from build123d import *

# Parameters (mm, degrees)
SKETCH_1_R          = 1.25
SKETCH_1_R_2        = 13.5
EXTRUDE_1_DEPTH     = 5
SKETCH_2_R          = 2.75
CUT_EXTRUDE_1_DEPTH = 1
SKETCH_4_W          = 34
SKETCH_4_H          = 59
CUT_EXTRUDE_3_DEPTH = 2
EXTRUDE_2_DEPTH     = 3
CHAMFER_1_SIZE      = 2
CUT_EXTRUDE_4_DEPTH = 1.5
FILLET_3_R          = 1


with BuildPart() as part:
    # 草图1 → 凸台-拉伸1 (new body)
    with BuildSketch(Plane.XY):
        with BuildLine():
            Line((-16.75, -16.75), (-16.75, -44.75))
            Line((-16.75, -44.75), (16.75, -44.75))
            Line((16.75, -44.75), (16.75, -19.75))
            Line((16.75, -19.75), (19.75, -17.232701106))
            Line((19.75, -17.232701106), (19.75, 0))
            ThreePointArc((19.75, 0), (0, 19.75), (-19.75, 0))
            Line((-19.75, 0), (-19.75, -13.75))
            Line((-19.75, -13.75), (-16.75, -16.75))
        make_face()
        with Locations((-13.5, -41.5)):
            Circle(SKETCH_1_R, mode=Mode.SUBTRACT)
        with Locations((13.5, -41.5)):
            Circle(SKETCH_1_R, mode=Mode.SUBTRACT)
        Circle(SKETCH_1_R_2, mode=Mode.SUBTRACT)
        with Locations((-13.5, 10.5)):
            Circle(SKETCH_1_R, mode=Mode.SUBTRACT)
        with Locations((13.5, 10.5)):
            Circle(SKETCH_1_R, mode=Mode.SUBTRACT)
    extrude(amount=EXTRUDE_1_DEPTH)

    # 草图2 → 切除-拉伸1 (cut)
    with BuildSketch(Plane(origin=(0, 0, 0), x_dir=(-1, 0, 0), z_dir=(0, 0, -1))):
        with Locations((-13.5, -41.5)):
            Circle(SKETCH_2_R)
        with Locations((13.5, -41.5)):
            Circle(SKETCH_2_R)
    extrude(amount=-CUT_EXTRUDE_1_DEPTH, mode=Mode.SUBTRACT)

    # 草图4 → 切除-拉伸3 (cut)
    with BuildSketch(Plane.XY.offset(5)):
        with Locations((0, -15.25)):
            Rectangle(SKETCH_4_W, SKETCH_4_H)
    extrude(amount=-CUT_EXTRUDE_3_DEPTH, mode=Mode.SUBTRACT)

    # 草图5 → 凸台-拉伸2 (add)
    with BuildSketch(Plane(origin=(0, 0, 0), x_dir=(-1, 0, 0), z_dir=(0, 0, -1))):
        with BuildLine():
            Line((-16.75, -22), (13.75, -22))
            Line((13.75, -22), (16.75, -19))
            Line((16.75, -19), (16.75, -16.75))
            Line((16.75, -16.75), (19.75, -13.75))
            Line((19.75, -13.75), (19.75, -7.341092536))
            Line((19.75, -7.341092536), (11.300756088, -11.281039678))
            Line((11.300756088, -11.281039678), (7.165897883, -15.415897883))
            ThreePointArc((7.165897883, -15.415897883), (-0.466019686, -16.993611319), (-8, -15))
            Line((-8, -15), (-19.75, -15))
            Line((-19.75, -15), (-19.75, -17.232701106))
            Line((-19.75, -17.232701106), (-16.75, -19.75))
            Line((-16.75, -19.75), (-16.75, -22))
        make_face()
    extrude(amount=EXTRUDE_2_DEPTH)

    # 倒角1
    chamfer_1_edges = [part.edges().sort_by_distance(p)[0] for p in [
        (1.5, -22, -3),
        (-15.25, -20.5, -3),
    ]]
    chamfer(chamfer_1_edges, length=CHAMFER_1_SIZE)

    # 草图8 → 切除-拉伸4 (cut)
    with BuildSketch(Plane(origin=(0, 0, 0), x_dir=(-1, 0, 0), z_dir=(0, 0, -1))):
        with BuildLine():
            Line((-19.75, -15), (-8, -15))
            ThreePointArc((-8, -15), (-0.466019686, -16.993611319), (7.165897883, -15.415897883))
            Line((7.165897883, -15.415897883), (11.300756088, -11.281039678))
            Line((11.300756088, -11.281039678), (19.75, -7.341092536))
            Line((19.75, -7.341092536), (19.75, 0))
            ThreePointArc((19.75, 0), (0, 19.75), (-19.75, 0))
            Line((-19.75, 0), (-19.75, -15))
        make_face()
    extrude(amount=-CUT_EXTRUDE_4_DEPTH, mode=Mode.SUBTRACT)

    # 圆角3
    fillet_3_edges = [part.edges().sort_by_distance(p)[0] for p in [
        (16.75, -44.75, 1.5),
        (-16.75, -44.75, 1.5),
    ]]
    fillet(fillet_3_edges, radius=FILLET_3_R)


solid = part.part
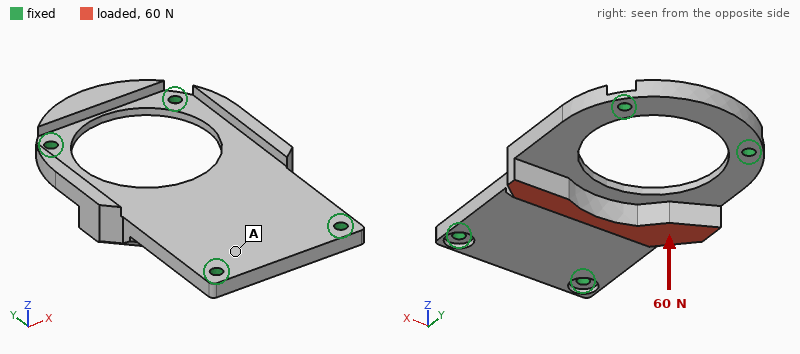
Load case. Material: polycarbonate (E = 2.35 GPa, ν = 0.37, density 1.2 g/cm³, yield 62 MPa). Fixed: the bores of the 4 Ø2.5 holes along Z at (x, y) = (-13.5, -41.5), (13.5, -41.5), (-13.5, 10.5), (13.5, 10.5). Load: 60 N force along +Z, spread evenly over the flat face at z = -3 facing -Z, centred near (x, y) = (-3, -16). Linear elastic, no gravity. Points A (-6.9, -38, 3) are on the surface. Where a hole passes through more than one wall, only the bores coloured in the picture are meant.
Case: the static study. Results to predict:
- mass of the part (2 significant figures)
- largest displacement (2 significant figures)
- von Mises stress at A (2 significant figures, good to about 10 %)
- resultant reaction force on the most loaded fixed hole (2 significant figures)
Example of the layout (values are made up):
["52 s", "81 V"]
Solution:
["6.2 g", "0.69 mm", "4.2 MPa", "19 N"]
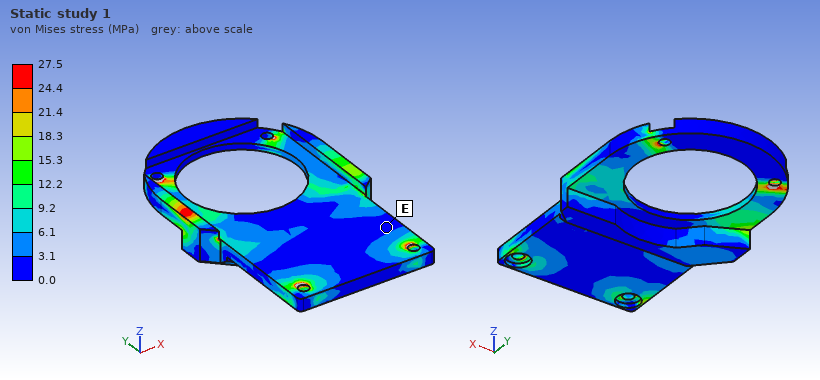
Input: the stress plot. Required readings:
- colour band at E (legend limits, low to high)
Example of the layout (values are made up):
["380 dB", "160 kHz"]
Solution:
["0.0 to 3.1 MPa"]
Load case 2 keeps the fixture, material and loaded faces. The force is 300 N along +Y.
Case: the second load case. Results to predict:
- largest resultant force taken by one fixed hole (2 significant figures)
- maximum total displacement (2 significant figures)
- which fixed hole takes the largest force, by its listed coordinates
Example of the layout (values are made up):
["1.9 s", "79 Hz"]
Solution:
["160 N", "0.69 mm", "(-13.5, -41.5)"]
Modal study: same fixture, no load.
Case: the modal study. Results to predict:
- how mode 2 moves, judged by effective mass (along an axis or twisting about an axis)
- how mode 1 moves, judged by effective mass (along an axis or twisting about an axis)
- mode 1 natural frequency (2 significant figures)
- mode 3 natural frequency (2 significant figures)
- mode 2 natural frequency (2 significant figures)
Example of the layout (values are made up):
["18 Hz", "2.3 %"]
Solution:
["twisting about Y", "along Z", "910 Hz", "2200 Hz", "1300 Hz"]
